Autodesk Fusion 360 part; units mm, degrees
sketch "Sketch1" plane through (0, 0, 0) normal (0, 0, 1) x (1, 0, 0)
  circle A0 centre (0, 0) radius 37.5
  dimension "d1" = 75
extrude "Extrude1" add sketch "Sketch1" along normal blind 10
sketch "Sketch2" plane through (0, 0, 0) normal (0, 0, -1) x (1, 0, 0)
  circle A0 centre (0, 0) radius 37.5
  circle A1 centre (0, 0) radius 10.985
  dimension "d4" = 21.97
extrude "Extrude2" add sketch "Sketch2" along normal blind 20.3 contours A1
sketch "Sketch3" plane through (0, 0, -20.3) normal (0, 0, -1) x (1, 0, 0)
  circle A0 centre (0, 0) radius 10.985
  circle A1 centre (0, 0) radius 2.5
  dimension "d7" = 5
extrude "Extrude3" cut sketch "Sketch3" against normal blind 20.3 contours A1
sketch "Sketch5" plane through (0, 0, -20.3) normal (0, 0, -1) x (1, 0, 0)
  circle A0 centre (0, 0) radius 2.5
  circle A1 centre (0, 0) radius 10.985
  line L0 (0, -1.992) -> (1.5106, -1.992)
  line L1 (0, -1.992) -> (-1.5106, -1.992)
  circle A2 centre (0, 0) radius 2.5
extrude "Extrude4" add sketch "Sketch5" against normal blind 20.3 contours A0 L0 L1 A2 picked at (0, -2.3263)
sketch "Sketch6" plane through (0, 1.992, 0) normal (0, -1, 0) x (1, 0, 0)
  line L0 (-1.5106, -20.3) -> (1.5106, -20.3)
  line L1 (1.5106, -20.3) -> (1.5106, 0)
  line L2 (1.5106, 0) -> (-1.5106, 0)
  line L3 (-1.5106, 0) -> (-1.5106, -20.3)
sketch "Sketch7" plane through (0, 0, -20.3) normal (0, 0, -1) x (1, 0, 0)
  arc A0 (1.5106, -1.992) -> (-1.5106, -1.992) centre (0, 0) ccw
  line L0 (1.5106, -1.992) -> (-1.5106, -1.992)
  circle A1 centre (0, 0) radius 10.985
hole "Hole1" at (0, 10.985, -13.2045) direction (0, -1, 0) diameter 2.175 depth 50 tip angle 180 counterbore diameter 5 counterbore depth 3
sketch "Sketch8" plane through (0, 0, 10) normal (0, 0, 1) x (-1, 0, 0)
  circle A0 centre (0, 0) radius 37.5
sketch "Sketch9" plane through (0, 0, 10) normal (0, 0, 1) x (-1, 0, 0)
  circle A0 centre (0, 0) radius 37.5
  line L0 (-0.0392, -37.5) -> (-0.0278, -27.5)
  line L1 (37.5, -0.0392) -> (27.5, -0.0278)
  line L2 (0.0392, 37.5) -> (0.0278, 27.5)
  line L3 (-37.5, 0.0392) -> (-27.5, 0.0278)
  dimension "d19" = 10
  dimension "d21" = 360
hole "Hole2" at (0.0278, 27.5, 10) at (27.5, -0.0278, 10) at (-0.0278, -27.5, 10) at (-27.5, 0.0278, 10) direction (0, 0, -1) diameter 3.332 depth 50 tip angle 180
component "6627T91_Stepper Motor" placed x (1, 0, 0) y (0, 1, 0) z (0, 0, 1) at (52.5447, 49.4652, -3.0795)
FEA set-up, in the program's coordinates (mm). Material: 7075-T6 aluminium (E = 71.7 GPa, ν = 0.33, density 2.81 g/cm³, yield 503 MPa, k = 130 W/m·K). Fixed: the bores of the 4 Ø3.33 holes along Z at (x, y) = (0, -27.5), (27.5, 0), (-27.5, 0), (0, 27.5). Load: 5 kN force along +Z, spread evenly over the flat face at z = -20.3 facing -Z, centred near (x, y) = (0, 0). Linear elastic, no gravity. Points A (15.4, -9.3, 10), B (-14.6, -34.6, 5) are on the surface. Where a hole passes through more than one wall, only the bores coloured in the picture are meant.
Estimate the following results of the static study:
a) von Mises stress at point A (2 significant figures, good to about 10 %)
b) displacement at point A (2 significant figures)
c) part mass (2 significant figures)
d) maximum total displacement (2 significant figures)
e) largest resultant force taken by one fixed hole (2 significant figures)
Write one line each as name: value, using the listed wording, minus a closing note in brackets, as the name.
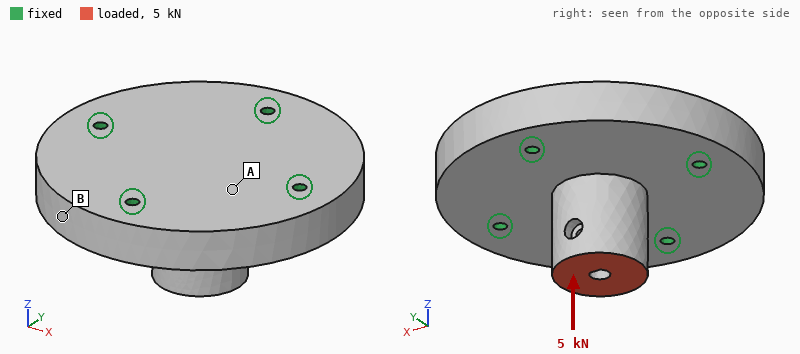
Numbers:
von Mises stress at point A: 13 MPa
displacement at point A: 7.5 µm
part mass: 140 g
maximum total displacement: 17 µm
largest resultant force taken by one fixed hole: 1.3 kN
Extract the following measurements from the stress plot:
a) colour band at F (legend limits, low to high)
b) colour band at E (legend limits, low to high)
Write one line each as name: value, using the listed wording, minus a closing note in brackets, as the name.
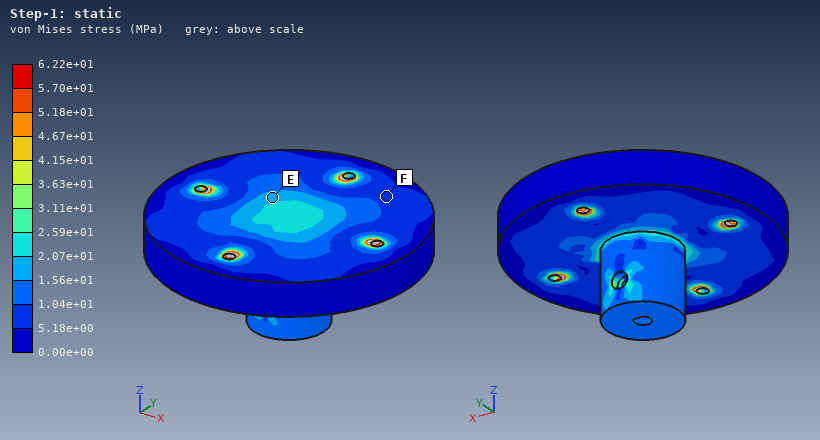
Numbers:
colour band at F: 5.18e+00 to 1.04e+01 MPa
colour band at E: 1.56e+01 to 2.07e+01 MPa
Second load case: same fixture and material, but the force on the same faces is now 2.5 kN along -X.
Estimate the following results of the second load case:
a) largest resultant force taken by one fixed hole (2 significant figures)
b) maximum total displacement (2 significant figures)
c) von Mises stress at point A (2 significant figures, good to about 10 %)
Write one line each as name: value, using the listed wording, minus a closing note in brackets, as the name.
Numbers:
largest resultant force taken by one fixed hole: 1.5 kN
maximum total displacement: 38 µm
von Mises stress at point A: 12 MPa
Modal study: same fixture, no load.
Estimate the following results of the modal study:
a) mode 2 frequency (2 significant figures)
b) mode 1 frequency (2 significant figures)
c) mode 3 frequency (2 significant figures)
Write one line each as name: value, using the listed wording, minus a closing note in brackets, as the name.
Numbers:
mode 2 frequency: 14 kHz
mode 1 frequency: 14 kHz
mode 3 frequency: 14 kHz
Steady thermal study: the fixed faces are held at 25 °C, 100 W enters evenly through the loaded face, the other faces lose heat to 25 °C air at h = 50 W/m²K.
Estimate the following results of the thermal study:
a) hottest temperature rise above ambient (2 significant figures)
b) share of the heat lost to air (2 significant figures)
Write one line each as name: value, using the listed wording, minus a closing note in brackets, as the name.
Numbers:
hottest temperature rise above ambient: 66 K
share of the heat lost to air: 7.3 %
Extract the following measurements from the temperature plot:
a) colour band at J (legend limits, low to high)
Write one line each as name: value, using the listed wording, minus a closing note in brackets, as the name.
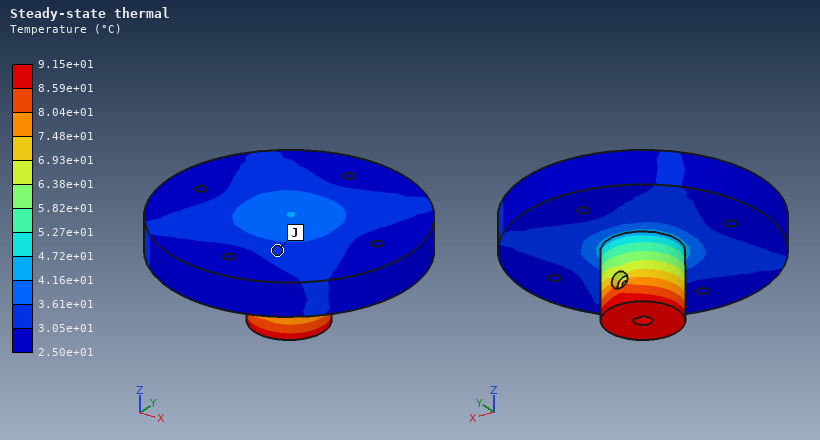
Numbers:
colour band at J: 3.05e+01 to 3.61e+01 °C
